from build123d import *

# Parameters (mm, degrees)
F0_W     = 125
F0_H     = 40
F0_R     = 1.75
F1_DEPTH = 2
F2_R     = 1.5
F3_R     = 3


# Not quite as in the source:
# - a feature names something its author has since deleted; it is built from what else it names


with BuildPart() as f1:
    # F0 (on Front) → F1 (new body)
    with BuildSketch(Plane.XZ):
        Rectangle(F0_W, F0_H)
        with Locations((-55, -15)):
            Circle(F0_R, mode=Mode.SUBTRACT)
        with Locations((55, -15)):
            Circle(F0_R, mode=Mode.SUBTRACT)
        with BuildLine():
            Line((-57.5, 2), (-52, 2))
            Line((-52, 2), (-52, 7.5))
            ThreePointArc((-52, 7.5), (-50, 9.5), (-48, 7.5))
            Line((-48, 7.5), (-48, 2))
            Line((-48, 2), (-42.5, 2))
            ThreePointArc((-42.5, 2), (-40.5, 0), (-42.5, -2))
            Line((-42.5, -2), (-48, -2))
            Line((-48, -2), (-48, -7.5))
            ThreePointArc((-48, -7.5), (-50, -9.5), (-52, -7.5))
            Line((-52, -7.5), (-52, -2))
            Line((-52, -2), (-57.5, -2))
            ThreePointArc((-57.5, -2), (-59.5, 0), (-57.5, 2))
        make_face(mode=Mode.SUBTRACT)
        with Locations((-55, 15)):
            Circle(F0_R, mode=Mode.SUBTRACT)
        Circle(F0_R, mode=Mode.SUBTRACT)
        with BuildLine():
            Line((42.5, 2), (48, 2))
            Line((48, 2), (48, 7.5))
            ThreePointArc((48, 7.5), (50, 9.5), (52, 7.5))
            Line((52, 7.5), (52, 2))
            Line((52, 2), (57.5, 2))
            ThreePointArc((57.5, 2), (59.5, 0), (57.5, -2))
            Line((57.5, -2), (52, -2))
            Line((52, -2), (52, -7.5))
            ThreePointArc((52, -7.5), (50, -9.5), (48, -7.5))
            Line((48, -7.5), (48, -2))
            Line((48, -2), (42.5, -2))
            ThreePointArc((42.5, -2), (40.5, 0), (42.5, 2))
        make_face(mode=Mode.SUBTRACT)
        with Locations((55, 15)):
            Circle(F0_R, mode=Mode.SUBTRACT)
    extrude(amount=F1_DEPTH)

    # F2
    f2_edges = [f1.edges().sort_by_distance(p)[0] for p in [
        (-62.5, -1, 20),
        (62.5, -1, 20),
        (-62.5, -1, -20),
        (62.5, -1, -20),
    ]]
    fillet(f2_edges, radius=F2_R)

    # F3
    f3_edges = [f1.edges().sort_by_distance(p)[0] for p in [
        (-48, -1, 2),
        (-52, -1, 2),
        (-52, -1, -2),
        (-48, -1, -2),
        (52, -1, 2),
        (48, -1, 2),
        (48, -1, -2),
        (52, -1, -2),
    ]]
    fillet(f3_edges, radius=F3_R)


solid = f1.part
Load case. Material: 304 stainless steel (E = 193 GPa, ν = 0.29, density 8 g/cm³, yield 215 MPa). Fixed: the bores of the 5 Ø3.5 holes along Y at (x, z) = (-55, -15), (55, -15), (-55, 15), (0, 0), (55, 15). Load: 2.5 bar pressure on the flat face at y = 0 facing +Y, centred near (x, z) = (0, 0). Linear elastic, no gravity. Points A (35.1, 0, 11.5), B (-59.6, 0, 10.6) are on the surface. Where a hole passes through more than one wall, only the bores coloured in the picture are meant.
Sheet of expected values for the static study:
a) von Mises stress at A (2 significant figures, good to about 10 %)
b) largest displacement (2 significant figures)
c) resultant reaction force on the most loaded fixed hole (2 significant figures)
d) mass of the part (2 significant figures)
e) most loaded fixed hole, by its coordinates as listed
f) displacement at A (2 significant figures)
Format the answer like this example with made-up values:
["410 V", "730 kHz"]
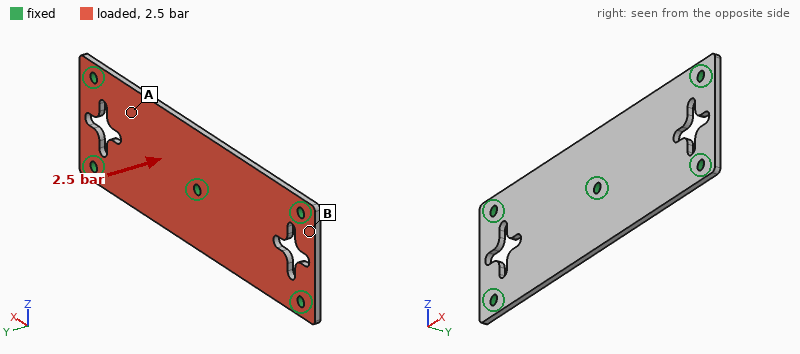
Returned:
["40 MPa", "64 µm", "560 N", "75 g", "(0, 0)", "46 µm"]
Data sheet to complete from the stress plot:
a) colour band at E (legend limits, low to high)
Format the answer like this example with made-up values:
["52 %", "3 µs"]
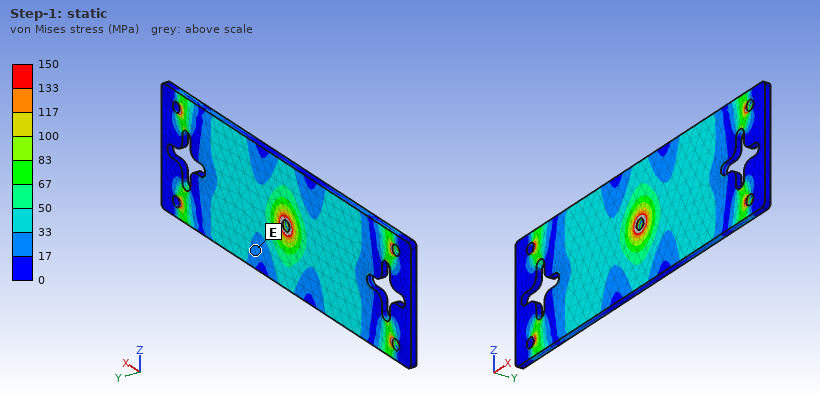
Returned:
["17 to 33 MPa"]
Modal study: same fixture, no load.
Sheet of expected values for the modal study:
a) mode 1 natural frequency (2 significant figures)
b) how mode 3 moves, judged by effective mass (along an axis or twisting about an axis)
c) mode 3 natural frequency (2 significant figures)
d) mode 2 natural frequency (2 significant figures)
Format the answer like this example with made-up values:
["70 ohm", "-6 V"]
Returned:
["2700 Hz", "along Y", "3000 Hz", "2800 Hz"]
